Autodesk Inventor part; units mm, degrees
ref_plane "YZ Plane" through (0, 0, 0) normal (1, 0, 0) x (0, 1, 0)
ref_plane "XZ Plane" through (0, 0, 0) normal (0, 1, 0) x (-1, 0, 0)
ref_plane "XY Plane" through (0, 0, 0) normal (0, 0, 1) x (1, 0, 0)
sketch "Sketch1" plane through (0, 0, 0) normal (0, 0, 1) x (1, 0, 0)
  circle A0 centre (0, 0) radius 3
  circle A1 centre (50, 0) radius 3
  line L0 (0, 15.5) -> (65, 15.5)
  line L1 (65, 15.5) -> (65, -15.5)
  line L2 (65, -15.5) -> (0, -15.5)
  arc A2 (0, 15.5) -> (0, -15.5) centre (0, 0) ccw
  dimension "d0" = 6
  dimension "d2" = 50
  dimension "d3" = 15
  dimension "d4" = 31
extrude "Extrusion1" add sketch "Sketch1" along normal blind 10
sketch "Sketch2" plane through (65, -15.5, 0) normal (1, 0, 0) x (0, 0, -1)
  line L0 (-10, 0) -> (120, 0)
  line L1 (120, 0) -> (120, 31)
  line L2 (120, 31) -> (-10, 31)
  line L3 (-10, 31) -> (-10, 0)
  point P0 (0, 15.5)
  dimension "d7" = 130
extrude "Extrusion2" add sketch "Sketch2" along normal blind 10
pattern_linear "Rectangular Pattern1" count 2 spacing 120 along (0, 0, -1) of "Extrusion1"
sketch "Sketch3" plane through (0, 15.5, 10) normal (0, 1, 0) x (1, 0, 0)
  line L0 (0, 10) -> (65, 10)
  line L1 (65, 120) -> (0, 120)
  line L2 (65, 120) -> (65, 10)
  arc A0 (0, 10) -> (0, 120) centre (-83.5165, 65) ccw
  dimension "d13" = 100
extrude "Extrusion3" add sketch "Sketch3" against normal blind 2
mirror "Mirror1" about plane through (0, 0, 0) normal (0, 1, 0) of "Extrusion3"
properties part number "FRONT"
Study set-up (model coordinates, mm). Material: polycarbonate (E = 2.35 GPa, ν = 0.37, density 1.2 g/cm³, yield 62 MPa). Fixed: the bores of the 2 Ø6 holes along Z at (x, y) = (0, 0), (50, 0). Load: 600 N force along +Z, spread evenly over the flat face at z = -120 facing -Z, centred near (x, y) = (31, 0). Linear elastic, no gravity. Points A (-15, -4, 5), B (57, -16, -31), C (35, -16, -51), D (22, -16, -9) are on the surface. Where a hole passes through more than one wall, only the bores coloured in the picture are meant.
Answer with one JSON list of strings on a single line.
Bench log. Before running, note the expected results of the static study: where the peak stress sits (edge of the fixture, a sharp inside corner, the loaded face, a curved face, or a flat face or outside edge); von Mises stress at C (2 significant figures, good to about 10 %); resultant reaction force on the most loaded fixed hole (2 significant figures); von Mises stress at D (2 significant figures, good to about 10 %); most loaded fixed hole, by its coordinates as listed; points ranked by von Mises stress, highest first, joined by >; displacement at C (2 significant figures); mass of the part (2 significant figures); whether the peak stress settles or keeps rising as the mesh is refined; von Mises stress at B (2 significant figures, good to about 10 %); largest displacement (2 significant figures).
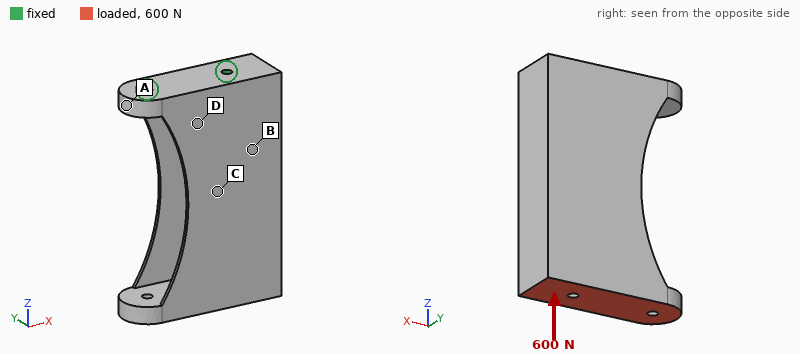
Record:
["edge of the fixture", "3.4 MPa", "360 N", "2.3 MPa", "(50, 0)", "C > D > B > A", "0.12 mm", "130 g", "keeps rising", "1.4 MPa", "0.65 mm"]
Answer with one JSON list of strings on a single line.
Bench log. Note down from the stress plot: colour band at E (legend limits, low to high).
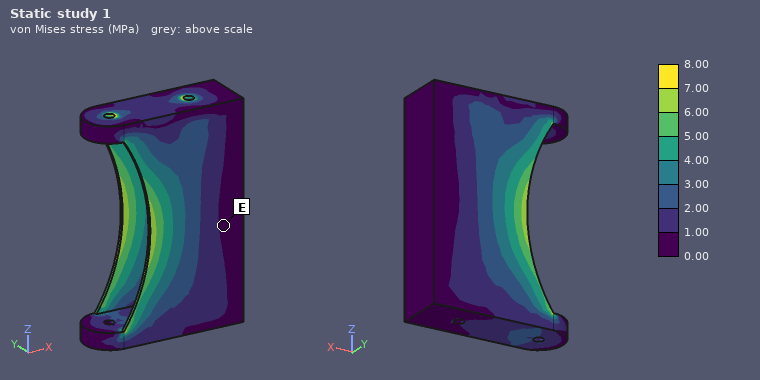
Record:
["0.00 to 1.00 MPa"]
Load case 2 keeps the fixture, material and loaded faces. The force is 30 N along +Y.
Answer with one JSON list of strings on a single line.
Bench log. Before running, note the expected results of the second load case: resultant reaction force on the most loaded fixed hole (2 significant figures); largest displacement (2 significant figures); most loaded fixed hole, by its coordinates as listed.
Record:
["20 N", "1.9 mm", "(50, 0)"]
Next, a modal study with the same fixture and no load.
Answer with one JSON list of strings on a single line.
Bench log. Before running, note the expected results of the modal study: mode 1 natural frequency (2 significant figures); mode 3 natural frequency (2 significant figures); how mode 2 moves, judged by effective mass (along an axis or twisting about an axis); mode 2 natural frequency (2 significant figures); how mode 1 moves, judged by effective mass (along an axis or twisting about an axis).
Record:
["110 Hz", "410 Hz", "along X", "340 Hz", "along Y"]
